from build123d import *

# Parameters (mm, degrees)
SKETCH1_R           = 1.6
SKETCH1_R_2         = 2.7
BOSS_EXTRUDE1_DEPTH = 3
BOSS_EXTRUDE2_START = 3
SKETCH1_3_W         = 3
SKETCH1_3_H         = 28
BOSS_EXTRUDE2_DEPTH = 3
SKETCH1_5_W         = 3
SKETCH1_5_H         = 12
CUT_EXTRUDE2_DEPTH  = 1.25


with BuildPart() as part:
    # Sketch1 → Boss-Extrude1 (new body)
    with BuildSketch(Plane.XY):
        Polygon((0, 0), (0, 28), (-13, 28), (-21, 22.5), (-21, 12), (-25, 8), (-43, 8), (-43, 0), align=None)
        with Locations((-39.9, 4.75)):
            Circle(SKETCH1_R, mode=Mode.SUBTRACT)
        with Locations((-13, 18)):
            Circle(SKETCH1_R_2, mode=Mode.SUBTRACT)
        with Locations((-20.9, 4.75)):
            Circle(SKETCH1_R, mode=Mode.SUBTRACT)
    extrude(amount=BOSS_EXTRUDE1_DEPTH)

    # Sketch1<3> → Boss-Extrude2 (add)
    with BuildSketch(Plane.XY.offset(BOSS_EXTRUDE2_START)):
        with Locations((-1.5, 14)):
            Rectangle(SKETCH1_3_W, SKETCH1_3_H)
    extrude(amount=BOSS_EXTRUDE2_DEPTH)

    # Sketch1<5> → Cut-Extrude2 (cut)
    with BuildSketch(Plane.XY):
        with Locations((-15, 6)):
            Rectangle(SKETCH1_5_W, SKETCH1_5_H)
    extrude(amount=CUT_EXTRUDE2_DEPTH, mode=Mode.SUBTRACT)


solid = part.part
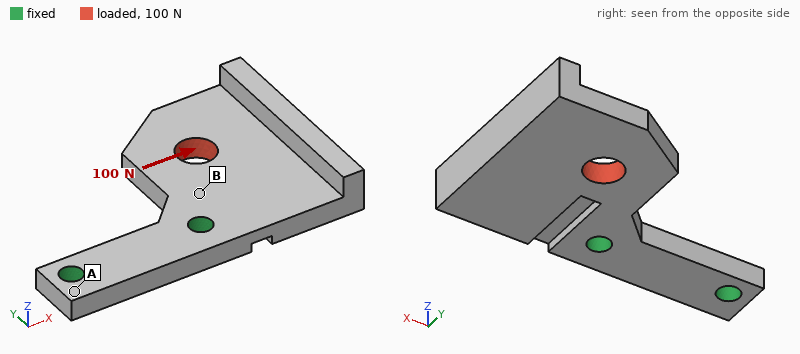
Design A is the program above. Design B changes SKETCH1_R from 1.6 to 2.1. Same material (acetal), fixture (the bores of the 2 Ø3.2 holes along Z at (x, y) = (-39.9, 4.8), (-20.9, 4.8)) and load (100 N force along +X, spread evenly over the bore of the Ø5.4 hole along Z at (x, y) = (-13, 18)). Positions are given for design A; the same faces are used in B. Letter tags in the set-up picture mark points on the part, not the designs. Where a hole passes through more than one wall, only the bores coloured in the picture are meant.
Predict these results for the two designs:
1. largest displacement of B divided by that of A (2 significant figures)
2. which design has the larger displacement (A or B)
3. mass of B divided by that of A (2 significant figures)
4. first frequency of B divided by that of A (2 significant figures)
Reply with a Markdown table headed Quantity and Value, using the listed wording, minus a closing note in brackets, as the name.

| Quantity | Value |
|---|---|
| largest displacement of B divided by that of A | 0.81 |
| which design has the larger displacement | A |
| mass of B divided by that of A | 0.99 |
| first frequency of B divided by that of A | 1.0 |
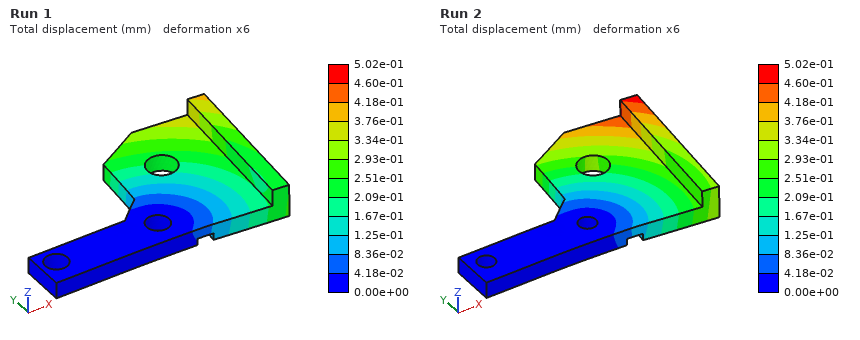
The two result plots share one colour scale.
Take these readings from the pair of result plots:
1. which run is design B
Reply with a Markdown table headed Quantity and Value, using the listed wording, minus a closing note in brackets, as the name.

| Quantity | Value |
|---|---|
| which run is design B | Run 1 |
